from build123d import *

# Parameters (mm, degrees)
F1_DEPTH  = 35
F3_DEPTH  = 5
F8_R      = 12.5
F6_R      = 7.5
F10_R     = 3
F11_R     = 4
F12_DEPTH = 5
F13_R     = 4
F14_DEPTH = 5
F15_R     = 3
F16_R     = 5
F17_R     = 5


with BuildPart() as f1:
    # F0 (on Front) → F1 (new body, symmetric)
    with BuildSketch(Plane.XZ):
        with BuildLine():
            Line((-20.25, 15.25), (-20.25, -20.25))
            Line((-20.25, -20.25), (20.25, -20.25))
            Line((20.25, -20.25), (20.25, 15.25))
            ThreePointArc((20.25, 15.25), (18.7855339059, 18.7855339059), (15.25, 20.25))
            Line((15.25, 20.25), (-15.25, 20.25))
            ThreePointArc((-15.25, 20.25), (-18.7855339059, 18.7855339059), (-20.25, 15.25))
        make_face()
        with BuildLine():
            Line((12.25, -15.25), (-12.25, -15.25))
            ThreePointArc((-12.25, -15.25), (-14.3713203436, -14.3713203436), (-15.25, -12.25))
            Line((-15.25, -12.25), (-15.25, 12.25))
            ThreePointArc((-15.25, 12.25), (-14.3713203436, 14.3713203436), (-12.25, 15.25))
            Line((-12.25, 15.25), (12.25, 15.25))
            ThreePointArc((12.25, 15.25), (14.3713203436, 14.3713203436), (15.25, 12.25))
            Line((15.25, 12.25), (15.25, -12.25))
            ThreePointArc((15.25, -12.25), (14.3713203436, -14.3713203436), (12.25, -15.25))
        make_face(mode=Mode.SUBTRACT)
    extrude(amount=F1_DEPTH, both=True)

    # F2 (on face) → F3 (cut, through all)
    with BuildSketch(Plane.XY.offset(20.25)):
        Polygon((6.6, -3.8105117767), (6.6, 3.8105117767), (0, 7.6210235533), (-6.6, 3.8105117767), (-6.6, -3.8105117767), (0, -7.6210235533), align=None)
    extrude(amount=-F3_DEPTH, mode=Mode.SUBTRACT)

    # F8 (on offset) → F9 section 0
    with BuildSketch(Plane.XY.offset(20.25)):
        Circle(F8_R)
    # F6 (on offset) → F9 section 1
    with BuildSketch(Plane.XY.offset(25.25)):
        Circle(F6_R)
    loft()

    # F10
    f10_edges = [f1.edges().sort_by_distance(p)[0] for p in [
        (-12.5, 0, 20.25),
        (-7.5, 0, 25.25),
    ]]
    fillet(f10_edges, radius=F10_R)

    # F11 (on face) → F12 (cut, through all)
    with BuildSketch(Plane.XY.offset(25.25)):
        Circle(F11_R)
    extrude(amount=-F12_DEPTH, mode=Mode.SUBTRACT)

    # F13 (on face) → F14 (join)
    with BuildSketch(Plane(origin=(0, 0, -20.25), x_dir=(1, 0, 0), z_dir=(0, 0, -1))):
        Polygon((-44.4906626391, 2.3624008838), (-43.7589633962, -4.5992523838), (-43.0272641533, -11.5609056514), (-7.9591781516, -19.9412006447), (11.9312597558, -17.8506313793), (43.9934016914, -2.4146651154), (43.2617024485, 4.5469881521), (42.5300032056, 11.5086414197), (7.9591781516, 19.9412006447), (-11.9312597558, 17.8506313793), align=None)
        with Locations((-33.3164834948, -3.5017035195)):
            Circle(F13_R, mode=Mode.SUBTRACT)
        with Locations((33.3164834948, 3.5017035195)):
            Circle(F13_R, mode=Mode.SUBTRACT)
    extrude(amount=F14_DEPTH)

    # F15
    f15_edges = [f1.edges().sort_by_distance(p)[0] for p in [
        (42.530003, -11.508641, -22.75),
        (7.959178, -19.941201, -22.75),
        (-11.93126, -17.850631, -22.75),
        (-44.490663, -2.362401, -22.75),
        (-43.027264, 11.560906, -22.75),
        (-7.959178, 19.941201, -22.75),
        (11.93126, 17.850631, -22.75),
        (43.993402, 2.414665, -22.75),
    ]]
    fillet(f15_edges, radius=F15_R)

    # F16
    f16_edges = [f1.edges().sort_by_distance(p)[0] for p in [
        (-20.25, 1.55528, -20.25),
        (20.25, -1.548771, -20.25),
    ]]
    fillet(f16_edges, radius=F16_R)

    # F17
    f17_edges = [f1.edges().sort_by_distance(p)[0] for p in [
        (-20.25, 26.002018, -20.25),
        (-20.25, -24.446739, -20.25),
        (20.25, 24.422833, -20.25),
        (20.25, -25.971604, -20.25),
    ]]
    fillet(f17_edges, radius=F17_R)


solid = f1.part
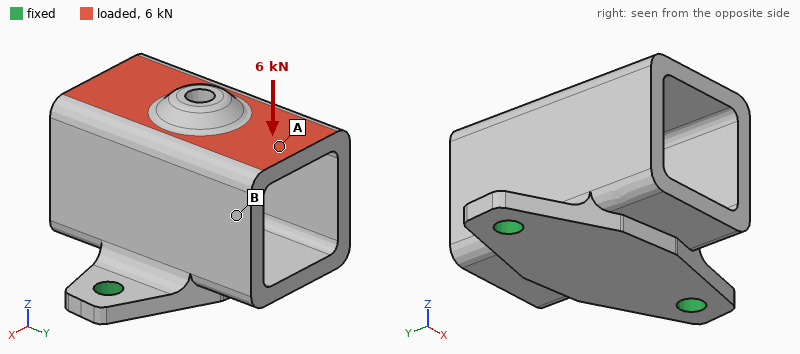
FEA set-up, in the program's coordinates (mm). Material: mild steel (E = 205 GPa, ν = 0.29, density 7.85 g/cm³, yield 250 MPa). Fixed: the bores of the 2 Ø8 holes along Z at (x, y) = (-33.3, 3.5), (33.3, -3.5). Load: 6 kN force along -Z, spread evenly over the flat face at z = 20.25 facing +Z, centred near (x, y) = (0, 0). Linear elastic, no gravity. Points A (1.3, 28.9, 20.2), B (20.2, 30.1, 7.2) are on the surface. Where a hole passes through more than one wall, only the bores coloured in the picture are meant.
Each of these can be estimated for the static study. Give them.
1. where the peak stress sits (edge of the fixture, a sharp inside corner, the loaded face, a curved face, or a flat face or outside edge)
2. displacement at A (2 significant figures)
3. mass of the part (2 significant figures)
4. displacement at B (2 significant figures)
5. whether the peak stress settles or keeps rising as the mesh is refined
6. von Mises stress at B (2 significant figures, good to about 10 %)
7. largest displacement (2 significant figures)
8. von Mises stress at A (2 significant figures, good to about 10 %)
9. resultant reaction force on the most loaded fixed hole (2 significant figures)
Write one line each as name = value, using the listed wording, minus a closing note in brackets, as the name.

where the peak stress sits = edge of the fixture
displacement at A = 28 µm
mass of the part = 490 g
displacement at B = 17 µm
whether the peak stress settles or keeps rising as the mesh is refined = keeps rising
von Mises stress at B = 20 MPa
largest displacement = 30 µm
von Mises stress at A = 54 MPa
resultant reaction force on the most loaded fixed hole = 3.5 kN
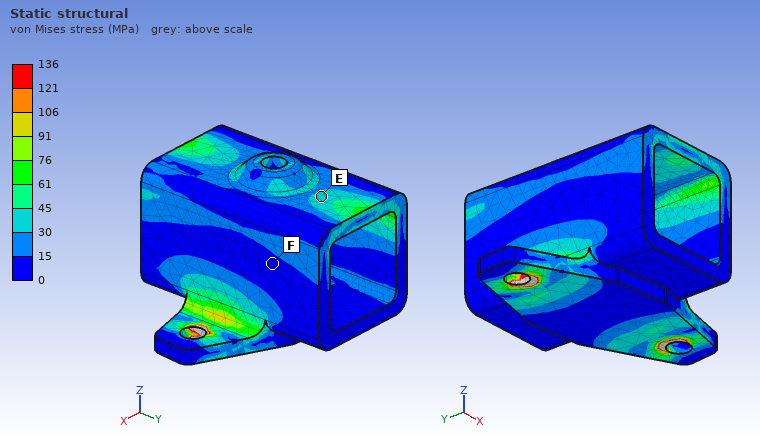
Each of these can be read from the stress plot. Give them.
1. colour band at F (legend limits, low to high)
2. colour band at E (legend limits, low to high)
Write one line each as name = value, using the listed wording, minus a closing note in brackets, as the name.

colour band at F = 0 to 15 MPa
colour band at E = 30 to 45 MPa
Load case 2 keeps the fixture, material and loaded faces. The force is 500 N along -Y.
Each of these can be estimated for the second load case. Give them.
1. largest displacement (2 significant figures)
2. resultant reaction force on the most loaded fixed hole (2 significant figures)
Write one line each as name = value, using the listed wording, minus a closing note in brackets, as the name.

largest displacement = 56 µm
resultant reaction force on the most loaded fixed hole = 250 N
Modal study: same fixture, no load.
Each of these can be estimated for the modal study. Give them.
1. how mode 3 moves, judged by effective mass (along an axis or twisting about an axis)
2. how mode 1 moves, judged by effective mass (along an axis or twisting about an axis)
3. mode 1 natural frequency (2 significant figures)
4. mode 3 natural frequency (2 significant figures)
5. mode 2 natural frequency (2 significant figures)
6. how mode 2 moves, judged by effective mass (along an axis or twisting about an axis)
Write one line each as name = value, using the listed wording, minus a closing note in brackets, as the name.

how mode 3 moves, judged by effective mass = along Z
how mode 1 moves, judged by effective mass = along Y
mode 1 natural frequency = 1100 Hz
mode 3 natural frequency = 4500 Hz
mode 2 natural frequency = 2800 Hz
how mode 2 moves, judged by effective mass = along X
